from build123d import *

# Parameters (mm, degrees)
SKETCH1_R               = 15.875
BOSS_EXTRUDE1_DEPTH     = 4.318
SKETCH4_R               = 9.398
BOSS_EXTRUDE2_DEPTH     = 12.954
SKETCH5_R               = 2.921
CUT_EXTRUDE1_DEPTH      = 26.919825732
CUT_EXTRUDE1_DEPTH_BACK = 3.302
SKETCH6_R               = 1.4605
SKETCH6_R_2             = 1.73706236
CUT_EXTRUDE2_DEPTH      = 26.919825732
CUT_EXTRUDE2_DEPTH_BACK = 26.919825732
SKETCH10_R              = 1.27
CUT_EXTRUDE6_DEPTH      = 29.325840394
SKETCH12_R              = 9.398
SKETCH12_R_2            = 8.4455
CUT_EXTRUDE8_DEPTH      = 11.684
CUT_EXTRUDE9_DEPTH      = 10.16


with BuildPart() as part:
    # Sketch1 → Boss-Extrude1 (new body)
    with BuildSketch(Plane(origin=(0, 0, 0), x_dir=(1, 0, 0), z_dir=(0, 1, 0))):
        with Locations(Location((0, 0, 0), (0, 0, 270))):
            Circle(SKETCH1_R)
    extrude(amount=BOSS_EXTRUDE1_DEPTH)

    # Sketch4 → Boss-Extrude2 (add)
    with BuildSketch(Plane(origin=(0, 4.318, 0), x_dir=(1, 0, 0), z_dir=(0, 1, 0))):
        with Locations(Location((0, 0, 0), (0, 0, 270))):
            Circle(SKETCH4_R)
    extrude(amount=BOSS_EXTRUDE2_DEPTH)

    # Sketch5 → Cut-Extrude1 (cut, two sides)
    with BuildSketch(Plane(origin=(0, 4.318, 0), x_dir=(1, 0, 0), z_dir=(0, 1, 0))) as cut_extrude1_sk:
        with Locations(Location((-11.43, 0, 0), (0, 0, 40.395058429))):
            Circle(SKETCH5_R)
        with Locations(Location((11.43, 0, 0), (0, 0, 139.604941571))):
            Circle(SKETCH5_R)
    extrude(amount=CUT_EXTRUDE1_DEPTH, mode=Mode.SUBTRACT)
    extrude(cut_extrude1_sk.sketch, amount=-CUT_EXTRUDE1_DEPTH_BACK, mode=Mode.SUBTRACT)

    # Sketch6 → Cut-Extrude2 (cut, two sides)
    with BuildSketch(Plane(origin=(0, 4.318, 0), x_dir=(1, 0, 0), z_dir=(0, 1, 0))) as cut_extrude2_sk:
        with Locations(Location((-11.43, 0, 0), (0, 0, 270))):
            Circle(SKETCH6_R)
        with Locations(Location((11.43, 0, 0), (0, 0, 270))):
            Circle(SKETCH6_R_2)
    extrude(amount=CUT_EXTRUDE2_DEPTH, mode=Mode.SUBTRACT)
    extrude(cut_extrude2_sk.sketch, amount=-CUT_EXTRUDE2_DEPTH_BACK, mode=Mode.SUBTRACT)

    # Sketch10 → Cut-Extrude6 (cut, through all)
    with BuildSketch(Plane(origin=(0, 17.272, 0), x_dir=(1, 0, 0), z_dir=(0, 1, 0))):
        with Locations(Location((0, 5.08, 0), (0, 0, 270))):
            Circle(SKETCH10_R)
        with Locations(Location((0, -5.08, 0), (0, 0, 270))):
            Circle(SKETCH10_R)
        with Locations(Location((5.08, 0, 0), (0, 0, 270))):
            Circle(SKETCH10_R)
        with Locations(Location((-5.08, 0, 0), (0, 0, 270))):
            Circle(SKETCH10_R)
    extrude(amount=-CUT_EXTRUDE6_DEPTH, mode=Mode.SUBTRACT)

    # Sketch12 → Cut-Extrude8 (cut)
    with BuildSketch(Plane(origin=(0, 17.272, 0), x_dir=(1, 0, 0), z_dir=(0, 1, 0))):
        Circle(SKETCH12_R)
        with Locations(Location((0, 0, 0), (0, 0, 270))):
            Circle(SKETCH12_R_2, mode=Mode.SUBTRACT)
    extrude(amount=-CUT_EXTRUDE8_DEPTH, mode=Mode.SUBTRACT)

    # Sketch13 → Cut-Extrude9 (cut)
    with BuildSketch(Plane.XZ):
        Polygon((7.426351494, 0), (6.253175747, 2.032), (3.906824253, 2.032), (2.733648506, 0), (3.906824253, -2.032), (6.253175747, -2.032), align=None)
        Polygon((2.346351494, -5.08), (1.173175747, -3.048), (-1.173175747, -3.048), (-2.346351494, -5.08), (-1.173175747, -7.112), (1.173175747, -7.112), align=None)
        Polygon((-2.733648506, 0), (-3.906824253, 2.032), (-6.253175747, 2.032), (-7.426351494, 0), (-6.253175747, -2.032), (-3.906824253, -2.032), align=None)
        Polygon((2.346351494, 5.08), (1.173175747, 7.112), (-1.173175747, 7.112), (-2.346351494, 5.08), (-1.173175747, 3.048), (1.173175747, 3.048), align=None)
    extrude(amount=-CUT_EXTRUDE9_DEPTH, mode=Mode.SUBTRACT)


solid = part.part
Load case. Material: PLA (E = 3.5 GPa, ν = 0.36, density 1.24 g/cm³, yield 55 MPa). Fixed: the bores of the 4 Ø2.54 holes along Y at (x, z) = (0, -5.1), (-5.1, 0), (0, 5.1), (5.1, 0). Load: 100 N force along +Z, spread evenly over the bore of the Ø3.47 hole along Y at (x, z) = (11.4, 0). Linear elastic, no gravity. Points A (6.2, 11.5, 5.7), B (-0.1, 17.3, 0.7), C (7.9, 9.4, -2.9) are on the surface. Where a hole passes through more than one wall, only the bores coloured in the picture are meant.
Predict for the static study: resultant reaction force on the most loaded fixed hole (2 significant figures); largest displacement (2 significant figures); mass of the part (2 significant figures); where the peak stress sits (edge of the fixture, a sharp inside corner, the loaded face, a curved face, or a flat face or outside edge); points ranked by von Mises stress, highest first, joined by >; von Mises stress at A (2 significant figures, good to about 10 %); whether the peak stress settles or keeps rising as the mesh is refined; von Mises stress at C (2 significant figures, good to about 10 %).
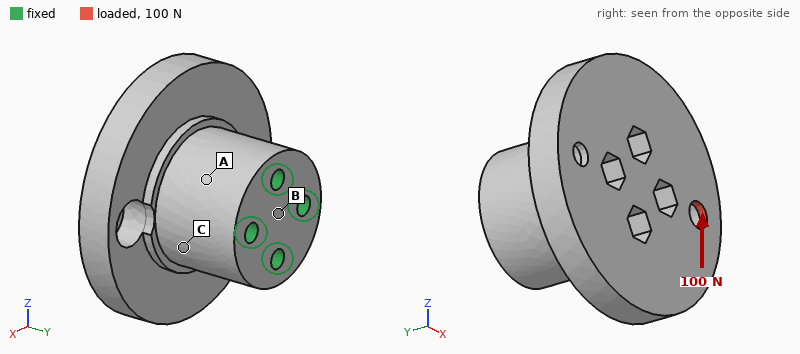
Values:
95 N
53 µm
6.8 g
a sharp inside corner
C > A > B
2.2 MPa
keeps rising
3.7 MPa
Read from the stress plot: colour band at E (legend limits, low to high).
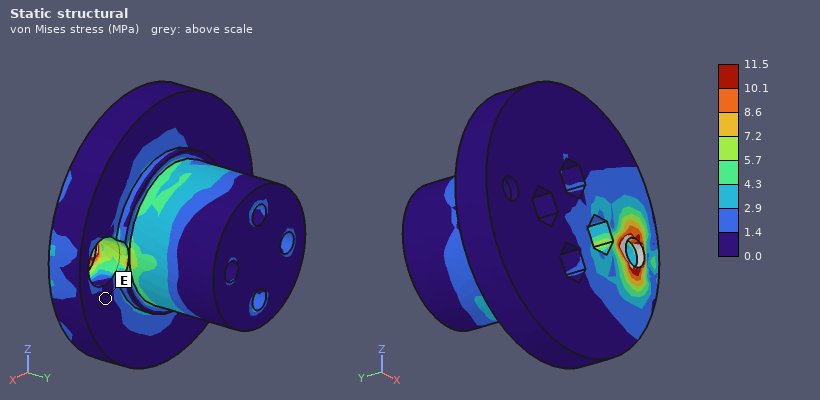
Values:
0.0 to 1.4 MPa
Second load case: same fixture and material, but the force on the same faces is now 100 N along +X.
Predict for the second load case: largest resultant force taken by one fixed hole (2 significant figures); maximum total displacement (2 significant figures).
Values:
84 N
54 µm
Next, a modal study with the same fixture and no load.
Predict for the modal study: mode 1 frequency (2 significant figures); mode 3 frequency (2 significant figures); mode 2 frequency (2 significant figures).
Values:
6000 Hz
6200 Hz
6100 Hz
